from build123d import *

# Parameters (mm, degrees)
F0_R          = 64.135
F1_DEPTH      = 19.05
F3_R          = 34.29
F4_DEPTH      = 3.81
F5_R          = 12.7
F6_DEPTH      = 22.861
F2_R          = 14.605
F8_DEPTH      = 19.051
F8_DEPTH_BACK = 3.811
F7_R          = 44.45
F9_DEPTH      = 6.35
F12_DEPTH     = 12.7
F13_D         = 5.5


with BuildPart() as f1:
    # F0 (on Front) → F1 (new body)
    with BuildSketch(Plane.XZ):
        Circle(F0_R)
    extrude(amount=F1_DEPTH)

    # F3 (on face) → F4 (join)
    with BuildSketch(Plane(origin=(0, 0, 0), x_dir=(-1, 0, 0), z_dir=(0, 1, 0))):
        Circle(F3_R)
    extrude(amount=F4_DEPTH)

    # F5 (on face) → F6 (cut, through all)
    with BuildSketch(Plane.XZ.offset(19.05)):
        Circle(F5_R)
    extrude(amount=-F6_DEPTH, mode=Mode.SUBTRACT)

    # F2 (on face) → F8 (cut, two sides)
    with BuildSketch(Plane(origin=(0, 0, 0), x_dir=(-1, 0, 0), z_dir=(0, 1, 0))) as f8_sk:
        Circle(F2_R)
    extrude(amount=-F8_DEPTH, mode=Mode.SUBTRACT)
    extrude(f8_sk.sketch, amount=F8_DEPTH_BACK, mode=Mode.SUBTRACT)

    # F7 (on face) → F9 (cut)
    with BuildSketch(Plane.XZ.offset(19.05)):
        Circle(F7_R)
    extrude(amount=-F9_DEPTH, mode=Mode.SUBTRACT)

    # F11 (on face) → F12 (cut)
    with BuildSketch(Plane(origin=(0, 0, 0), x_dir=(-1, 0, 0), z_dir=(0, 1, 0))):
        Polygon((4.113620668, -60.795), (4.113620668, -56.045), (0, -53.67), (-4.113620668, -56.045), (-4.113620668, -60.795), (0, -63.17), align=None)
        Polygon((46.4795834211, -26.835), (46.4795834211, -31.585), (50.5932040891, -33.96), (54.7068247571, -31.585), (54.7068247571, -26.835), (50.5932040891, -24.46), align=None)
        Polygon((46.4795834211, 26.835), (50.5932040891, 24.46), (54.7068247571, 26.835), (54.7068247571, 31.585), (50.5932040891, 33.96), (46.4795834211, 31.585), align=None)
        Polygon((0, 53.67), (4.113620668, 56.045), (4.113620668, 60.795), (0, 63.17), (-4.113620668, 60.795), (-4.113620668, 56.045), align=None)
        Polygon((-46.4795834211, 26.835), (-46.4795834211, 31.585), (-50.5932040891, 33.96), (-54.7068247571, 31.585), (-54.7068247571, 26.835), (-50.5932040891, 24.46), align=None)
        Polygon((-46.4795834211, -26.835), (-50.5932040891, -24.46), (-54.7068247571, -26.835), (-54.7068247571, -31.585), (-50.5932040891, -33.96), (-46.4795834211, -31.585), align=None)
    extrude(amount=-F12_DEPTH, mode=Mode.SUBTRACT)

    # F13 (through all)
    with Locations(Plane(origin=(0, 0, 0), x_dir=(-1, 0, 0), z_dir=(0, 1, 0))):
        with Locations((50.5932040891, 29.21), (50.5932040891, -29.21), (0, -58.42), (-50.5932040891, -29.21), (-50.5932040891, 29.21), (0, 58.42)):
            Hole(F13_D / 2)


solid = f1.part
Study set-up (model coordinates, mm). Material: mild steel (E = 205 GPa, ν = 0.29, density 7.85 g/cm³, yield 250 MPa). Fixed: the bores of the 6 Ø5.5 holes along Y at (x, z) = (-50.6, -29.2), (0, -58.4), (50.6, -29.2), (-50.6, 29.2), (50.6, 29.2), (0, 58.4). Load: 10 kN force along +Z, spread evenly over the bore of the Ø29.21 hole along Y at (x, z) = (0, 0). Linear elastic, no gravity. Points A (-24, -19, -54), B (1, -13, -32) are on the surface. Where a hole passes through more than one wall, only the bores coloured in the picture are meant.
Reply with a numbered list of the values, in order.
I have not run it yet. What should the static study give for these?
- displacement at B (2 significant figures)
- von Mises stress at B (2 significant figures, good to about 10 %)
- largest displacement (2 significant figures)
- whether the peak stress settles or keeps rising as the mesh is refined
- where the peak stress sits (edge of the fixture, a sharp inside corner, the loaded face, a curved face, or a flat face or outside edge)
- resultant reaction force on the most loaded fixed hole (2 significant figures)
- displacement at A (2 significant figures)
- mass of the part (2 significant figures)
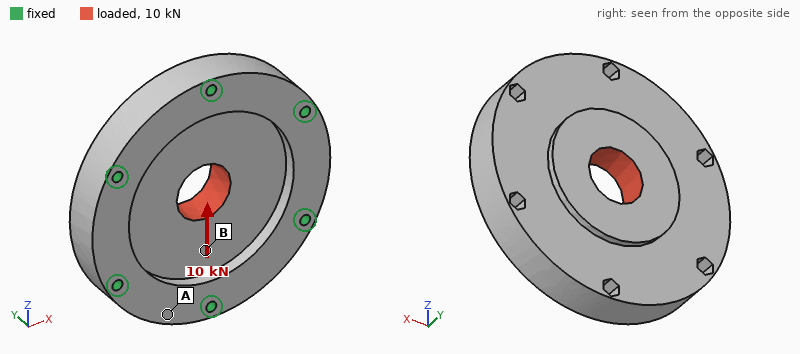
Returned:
1. 1.9 µm
2. 8.1 MPa
3. 2.5 µm
4. keeps rising
5. edge of the fixture
6. 2.0 kN
7. 0.88 µm
8. 1.6 kg
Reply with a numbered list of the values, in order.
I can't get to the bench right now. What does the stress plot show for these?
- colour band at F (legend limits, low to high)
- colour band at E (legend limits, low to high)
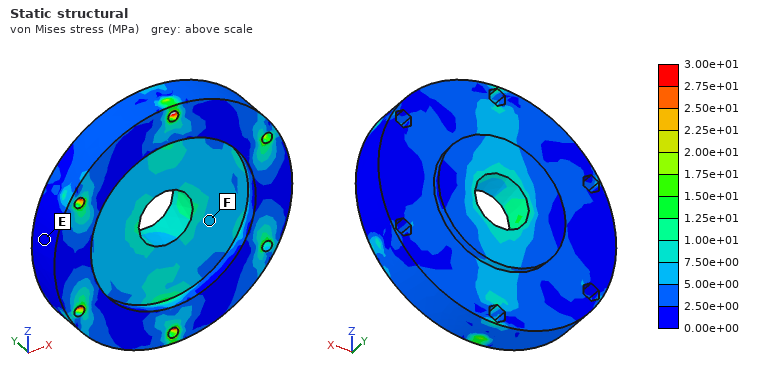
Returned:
1. 5.00e+00 to 7.50e+00 MPa
2. 0.00e+00 to 2.50e+00 MPa
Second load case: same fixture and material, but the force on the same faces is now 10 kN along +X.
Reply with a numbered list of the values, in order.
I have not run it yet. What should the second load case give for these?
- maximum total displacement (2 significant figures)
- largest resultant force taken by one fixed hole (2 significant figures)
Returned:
1. 2.6 µm
2. 1.9 kN
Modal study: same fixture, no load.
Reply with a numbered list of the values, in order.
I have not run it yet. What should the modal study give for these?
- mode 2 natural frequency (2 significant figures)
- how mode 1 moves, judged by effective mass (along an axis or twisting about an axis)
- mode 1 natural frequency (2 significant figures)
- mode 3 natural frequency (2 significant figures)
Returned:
1. 11 kHz
2. along Y
3. 7600 Hz
4. 11 kHz
